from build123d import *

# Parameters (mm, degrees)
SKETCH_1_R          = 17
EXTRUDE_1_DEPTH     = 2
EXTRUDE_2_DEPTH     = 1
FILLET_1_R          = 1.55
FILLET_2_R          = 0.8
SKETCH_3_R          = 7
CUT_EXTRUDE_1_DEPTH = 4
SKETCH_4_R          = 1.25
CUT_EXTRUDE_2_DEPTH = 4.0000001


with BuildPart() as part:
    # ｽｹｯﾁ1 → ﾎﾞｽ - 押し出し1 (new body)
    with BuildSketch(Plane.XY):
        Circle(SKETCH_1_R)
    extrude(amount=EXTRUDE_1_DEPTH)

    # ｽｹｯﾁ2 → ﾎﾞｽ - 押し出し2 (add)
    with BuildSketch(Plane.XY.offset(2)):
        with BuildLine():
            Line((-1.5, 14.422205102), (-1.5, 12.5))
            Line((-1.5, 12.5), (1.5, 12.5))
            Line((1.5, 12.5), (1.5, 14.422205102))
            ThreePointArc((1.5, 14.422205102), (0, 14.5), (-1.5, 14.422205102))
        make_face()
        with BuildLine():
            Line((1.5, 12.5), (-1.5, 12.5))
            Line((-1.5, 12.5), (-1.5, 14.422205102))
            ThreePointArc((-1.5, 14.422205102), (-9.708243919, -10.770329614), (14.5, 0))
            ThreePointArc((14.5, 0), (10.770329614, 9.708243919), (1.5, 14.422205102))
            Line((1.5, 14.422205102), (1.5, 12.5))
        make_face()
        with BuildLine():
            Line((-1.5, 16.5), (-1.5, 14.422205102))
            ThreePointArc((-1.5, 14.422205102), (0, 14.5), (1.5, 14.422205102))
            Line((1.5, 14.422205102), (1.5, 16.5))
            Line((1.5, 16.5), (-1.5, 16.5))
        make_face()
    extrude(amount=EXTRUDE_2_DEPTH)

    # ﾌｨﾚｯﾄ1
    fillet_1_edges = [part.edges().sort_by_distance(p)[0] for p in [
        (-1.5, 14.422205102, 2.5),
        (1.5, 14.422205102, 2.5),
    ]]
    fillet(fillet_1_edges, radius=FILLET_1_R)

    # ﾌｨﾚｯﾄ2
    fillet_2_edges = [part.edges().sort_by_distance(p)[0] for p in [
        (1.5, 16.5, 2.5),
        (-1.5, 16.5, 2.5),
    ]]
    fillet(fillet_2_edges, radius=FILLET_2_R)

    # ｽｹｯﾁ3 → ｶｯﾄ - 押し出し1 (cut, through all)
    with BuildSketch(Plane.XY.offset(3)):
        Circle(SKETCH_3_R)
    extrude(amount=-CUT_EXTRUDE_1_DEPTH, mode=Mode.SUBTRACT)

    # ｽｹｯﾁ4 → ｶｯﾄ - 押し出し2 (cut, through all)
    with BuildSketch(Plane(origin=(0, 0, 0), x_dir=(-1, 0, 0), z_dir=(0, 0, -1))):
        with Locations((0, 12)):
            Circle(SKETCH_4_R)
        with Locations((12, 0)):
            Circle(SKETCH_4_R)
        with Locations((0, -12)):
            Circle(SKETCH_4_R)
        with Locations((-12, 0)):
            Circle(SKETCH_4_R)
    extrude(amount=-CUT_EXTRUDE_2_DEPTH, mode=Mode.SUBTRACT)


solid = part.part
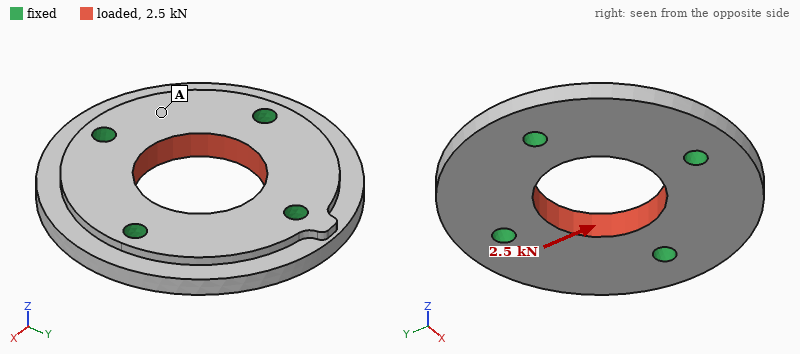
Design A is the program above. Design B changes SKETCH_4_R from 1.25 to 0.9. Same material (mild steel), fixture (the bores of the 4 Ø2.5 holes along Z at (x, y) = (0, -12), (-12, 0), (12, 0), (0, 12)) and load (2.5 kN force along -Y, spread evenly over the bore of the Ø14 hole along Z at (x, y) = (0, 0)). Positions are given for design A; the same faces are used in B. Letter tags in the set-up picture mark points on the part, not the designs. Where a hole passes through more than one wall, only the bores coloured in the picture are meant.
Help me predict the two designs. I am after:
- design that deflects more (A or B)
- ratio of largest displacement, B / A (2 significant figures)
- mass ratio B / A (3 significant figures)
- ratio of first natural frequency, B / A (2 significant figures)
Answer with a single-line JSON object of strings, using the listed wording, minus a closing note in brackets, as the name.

{"design that deflects more": "B", "ratio of largest displacement, B / A": "1.1", "mass ratio B / A": "1.01", "ratio of first natural frequency, B / A": "0.88"}
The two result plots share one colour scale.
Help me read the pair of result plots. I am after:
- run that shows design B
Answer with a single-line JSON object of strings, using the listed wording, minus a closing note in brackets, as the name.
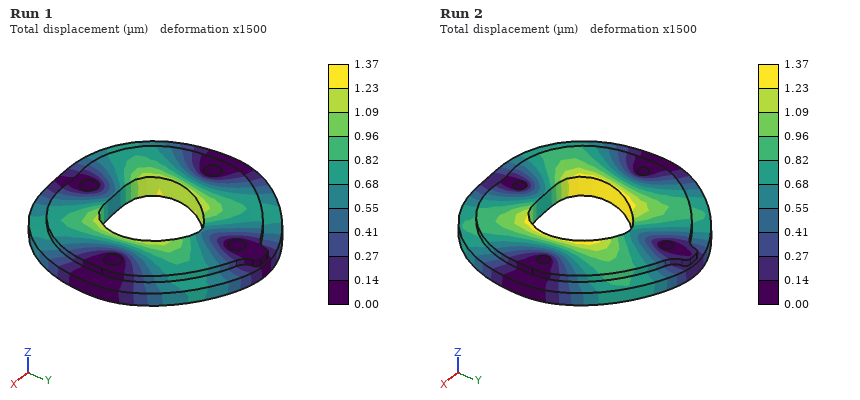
{"run that shows design B": "Run 2"}
